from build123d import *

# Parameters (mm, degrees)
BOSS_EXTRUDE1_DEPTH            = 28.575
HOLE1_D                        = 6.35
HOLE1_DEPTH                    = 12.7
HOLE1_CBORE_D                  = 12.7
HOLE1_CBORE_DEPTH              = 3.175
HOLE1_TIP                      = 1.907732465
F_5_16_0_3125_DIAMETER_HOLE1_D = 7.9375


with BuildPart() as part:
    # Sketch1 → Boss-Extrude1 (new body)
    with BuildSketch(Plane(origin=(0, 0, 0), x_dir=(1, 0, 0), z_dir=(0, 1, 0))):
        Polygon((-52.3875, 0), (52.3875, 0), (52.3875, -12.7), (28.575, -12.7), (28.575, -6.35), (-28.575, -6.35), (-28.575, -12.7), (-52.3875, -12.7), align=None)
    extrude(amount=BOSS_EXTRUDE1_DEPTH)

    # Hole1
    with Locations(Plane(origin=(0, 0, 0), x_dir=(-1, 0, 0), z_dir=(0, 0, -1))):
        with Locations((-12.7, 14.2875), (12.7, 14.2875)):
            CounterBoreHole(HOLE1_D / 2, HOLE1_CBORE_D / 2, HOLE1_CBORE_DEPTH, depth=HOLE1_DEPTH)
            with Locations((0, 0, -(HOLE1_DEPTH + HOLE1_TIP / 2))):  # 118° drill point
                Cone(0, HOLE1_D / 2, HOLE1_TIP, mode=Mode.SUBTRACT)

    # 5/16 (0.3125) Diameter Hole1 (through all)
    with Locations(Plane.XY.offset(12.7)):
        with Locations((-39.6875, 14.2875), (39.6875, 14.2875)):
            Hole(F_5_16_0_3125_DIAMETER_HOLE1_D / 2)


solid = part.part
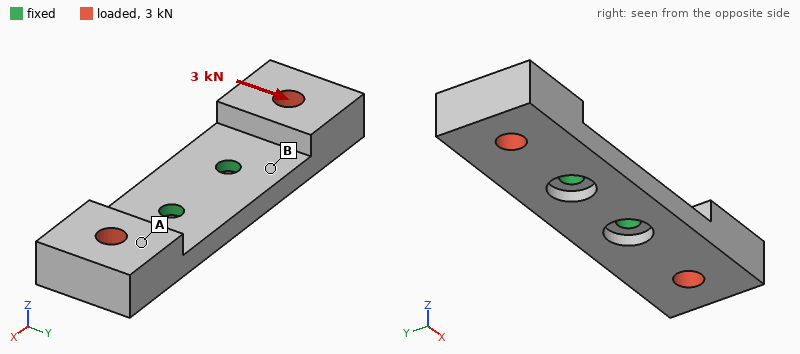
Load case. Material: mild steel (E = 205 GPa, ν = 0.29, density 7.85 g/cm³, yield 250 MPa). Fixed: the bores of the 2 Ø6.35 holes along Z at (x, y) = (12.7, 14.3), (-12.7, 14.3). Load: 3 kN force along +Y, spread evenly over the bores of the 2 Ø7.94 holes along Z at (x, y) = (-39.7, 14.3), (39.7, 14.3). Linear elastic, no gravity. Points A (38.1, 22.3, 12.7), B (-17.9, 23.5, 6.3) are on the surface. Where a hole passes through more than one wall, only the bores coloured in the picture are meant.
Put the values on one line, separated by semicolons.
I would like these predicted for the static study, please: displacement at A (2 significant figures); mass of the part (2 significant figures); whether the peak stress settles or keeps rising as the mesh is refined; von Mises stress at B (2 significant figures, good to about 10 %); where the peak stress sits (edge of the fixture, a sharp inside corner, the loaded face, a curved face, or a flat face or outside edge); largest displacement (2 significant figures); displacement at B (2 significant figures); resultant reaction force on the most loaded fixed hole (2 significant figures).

15 µm; 200 g; keeps rising; 32 MPa; edge of the fixture; 22 µm; 3.7 µm; 1.5 kN
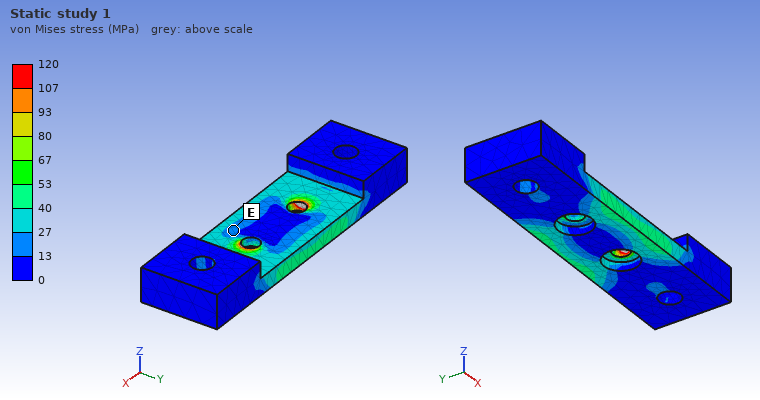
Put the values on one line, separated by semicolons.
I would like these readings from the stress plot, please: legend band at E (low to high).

13 to 27 MPa
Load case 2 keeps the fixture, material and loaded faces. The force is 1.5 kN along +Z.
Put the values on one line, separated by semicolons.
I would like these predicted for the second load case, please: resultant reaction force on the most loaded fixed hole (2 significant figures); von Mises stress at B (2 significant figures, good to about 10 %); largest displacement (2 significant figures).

2.2 kN; 80 MPa; 0.10 mm
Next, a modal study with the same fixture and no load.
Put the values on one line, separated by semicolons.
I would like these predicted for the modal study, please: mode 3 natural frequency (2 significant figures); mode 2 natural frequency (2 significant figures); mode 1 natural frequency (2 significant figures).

4700 Hz; 2000 Hz; 1900 Hz
